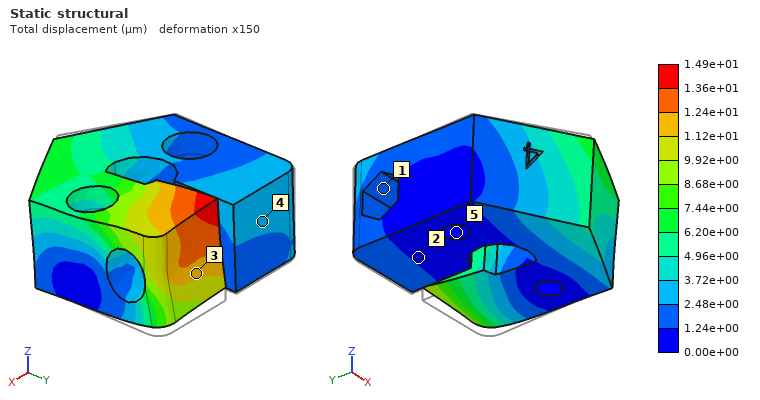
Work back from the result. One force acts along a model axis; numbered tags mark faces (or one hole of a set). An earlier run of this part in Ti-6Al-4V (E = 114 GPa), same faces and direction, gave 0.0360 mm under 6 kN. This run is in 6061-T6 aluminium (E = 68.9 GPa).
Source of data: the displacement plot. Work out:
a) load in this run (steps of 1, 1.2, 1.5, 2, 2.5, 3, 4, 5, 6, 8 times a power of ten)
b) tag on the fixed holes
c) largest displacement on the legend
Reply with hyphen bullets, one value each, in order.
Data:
- 1.5 kN
- 5
- 1.49e+01 µm
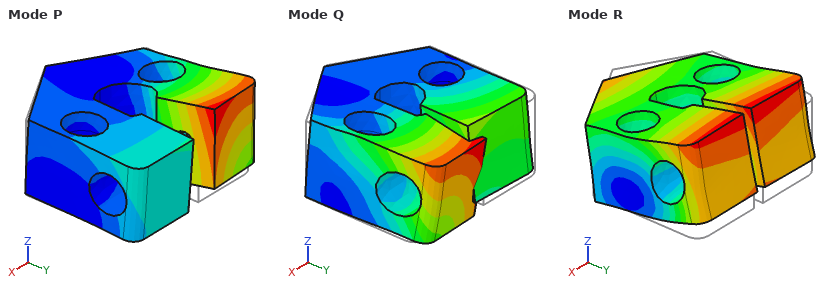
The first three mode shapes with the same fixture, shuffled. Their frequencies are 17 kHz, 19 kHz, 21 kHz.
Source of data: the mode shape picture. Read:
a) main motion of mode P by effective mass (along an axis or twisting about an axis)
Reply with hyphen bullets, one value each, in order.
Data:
- along X
